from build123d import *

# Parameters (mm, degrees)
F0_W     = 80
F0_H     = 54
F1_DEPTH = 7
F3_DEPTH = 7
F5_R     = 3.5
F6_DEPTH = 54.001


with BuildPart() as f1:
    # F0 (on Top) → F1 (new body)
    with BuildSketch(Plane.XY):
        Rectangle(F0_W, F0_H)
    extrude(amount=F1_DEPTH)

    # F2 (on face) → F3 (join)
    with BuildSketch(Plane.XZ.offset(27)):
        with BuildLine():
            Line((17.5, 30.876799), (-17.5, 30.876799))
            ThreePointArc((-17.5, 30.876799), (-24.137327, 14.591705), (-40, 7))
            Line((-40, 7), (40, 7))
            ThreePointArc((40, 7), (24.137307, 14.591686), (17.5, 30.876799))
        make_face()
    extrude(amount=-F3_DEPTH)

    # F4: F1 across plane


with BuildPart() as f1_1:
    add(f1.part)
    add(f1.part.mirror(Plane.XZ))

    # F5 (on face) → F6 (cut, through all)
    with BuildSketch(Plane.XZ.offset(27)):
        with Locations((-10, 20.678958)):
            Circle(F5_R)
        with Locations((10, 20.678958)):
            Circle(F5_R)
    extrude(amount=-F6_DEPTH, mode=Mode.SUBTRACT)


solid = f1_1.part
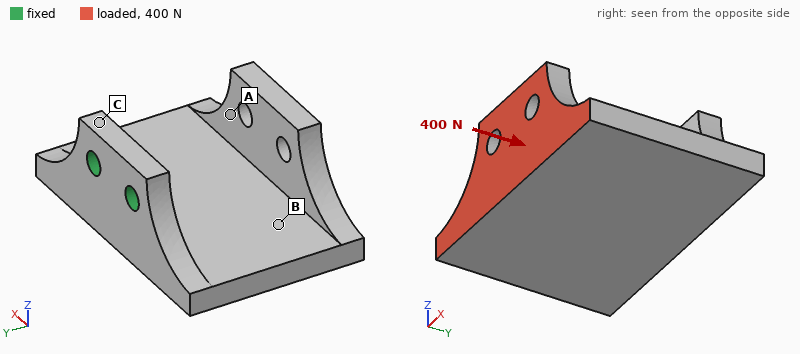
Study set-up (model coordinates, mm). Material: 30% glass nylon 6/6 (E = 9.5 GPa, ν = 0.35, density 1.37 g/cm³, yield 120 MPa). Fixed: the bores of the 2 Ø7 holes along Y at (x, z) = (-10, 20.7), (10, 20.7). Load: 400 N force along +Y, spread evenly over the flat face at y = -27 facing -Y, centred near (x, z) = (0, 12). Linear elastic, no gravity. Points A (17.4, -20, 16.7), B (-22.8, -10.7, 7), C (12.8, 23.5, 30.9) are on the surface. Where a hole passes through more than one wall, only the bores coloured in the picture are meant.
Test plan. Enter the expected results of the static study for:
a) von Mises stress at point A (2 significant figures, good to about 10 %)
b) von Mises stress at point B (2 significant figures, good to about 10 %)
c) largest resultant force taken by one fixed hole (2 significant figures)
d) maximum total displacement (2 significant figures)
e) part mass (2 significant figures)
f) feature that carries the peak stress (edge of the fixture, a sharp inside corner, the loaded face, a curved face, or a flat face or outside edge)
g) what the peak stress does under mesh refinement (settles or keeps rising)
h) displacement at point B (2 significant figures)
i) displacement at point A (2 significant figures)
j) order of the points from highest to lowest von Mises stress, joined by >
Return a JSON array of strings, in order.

["3.6 MPa", "5.5 MPa", "200 N", "0.31 mm", "61 g", "edge of the fixture", "keeps rising", "0.087 mm", "0.17 mm", "B > A > C"]
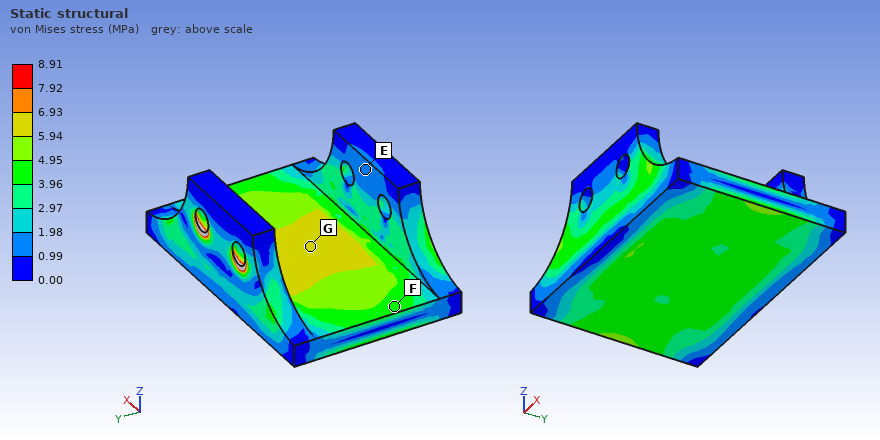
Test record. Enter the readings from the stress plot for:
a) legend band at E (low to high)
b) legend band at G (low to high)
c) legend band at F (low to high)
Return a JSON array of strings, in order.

["0.99 to 1.98 MPa", "5.94 to 6.93 MPa", "3.96 to 4.95 MPa"]
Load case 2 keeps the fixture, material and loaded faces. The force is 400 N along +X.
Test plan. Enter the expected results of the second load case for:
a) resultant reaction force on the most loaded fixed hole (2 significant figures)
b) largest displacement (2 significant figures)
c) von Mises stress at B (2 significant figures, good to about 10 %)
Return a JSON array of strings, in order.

["710 N", "0.58 mm", "6.5 MPa"]
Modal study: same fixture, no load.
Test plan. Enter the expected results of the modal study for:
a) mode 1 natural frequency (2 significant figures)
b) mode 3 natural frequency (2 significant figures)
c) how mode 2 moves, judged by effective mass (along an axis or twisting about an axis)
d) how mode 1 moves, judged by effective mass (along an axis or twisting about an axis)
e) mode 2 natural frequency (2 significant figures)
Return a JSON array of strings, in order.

["520 Hz", "1500 Hz", "along X", "along Z", "890 Hz"]
